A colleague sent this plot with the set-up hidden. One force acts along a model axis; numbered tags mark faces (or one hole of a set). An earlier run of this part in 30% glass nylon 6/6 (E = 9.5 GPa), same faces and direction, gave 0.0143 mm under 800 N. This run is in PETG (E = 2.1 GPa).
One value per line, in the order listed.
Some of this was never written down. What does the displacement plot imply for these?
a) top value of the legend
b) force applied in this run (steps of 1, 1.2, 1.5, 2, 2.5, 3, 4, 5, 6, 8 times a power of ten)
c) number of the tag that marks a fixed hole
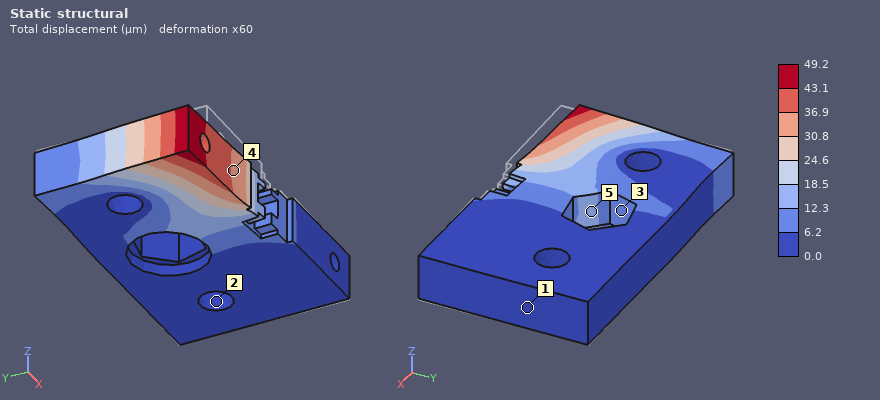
49.2 µm
600 N
2
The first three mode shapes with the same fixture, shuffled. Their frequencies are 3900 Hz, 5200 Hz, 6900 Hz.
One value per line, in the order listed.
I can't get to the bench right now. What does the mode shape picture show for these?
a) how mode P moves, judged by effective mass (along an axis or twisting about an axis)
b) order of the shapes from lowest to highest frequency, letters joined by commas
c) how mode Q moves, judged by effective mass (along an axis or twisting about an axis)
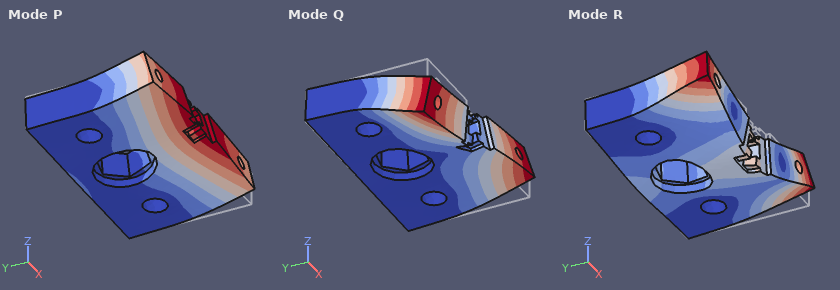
along Z
P, Q, R
twisting about Y
